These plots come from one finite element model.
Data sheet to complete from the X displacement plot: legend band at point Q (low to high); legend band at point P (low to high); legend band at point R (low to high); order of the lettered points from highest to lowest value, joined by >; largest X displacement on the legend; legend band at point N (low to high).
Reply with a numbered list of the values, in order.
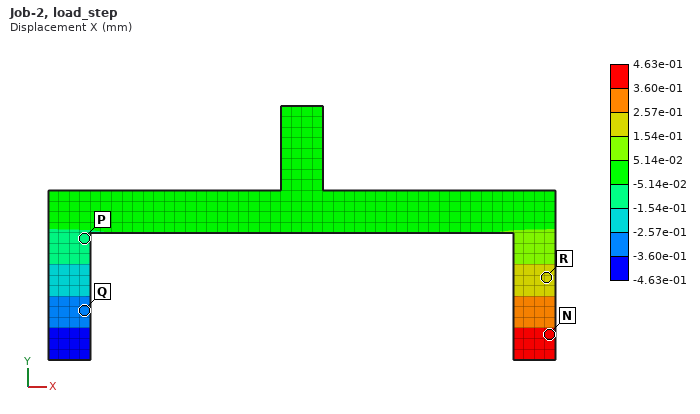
1. -3.60e-01 to -2.57e-01 mm
2. -1.54e-01 to -5.14e-02 mm
3. 1.54e-01 to 2.57e-01 mm
4. N > R > P > Q
5. 4.63e-01 mm
6. 3.60e-01 to 4.63e-01 mm
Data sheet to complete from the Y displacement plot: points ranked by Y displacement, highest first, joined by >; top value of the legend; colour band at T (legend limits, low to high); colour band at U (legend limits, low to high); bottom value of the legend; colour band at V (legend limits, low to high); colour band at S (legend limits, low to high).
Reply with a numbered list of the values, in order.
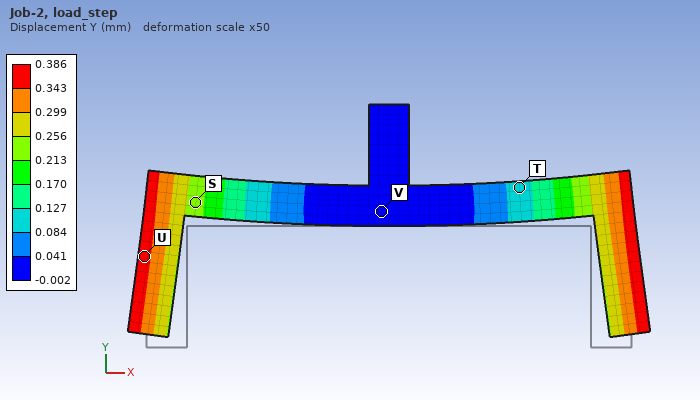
1. U > S > T > V
2. 0.386 mm
3. 0.084 to 0.127 mm
4. 0.343 to 0.386 mm
5. -0.002 mm
6. -0.002 to 0.041 mm
7. 0.213 to 0.256 mm
